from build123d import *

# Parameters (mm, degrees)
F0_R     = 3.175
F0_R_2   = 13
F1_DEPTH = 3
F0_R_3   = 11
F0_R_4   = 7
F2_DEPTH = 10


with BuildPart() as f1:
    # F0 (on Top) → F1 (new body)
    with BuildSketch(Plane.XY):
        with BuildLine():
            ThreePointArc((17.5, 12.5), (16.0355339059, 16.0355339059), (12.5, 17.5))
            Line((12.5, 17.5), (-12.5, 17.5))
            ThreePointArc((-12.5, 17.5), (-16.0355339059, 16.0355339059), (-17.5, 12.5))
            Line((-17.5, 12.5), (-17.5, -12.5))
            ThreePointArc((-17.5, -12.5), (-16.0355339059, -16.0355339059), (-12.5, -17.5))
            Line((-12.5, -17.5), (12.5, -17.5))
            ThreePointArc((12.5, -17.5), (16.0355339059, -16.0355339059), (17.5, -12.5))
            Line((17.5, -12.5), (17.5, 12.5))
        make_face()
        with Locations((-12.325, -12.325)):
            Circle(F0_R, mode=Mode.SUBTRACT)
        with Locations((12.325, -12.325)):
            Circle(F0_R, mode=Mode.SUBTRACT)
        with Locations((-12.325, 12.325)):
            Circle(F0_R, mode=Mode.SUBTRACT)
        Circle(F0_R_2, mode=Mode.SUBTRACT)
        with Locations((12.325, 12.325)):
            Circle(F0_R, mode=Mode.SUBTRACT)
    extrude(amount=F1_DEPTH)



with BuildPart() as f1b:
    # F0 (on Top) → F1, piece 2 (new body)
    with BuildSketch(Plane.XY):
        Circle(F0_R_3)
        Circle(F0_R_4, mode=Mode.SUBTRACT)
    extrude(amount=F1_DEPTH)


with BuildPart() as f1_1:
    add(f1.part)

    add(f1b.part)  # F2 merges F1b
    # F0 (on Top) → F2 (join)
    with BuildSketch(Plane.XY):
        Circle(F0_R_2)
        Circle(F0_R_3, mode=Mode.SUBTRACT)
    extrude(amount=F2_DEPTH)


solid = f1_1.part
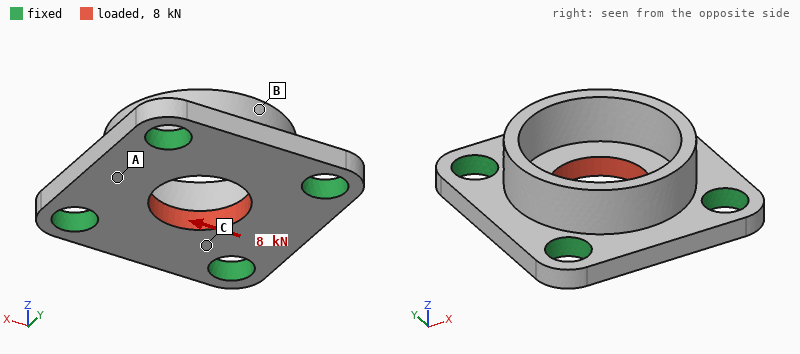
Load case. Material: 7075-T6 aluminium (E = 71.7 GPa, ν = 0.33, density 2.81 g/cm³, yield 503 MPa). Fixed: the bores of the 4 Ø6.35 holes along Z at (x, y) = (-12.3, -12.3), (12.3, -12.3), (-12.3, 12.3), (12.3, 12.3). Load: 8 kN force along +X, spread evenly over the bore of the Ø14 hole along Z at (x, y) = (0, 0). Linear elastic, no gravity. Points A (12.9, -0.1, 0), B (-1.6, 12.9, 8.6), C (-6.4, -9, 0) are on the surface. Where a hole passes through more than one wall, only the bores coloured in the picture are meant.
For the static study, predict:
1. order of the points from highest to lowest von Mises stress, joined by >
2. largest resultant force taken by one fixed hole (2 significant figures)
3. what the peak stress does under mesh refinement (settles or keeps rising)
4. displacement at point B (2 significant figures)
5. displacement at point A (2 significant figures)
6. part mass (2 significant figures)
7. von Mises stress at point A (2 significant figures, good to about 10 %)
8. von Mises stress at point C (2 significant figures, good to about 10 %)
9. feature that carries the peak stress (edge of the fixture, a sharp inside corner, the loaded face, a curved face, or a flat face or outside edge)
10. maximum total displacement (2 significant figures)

C > A > B
2.1 kN
keeps rising
3.7 µm
12 µm
11 g
27 MPa
65 MPa
edge of the fixture
15 µm
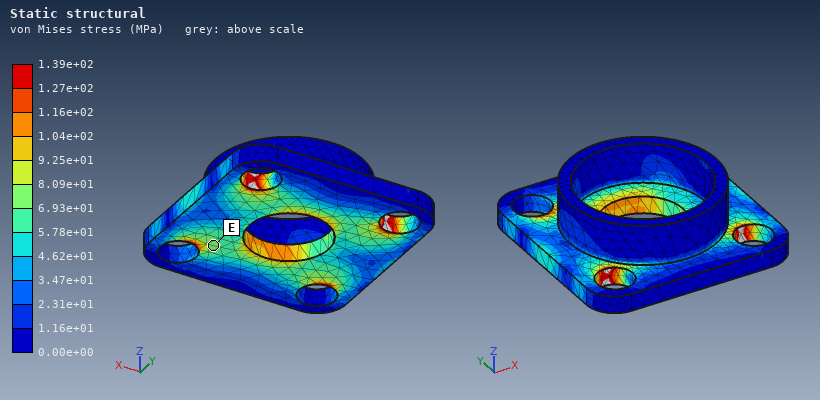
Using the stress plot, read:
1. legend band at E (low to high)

6.93e+01 to 8.09e+01 MPa
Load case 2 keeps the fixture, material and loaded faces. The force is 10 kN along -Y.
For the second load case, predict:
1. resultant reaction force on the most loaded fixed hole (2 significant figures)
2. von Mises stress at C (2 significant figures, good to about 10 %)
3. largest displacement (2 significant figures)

2.6 kN
89 MPa
19 µm
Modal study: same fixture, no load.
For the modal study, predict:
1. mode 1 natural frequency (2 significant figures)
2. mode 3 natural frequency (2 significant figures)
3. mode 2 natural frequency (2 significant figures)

29 kHz
35 kHz
35 kHz
